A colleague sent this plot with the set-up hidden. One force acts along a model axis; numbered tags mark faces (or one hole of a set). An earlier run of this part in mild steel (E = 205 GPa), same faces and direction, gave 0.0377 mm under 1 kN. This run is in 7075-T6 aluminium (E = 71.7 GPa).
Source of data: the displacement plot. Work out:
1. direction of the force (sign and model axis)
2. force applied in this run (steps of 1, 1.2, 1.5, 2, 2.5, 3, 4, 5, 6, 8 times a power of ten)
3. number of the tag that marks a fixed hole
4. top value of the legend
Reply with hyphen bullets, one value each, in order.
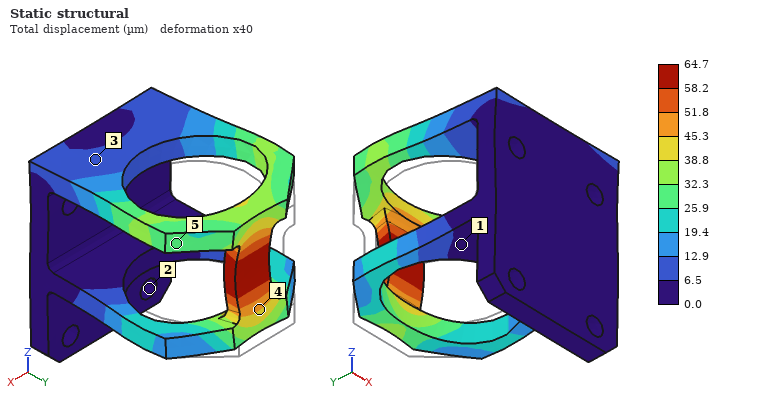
- -Y
- 600 N
- 2
- 64.7 µm
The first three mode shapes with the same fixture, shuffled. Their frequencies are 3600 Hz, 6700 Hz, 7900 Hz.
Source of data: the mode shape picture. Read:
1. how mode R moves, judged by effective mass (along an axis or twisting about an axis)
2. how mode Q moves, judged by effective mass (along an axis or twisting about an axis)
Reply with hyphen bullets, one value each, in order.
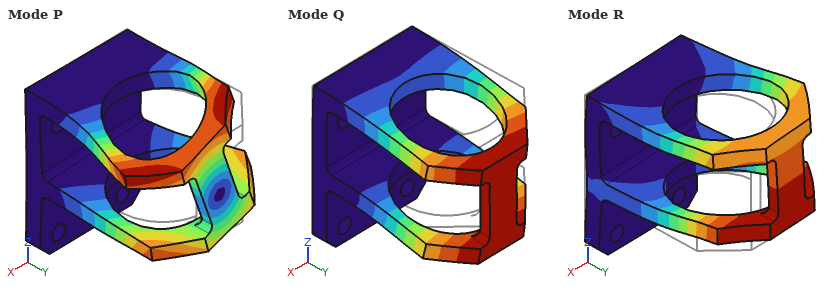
- along X
- along Z
